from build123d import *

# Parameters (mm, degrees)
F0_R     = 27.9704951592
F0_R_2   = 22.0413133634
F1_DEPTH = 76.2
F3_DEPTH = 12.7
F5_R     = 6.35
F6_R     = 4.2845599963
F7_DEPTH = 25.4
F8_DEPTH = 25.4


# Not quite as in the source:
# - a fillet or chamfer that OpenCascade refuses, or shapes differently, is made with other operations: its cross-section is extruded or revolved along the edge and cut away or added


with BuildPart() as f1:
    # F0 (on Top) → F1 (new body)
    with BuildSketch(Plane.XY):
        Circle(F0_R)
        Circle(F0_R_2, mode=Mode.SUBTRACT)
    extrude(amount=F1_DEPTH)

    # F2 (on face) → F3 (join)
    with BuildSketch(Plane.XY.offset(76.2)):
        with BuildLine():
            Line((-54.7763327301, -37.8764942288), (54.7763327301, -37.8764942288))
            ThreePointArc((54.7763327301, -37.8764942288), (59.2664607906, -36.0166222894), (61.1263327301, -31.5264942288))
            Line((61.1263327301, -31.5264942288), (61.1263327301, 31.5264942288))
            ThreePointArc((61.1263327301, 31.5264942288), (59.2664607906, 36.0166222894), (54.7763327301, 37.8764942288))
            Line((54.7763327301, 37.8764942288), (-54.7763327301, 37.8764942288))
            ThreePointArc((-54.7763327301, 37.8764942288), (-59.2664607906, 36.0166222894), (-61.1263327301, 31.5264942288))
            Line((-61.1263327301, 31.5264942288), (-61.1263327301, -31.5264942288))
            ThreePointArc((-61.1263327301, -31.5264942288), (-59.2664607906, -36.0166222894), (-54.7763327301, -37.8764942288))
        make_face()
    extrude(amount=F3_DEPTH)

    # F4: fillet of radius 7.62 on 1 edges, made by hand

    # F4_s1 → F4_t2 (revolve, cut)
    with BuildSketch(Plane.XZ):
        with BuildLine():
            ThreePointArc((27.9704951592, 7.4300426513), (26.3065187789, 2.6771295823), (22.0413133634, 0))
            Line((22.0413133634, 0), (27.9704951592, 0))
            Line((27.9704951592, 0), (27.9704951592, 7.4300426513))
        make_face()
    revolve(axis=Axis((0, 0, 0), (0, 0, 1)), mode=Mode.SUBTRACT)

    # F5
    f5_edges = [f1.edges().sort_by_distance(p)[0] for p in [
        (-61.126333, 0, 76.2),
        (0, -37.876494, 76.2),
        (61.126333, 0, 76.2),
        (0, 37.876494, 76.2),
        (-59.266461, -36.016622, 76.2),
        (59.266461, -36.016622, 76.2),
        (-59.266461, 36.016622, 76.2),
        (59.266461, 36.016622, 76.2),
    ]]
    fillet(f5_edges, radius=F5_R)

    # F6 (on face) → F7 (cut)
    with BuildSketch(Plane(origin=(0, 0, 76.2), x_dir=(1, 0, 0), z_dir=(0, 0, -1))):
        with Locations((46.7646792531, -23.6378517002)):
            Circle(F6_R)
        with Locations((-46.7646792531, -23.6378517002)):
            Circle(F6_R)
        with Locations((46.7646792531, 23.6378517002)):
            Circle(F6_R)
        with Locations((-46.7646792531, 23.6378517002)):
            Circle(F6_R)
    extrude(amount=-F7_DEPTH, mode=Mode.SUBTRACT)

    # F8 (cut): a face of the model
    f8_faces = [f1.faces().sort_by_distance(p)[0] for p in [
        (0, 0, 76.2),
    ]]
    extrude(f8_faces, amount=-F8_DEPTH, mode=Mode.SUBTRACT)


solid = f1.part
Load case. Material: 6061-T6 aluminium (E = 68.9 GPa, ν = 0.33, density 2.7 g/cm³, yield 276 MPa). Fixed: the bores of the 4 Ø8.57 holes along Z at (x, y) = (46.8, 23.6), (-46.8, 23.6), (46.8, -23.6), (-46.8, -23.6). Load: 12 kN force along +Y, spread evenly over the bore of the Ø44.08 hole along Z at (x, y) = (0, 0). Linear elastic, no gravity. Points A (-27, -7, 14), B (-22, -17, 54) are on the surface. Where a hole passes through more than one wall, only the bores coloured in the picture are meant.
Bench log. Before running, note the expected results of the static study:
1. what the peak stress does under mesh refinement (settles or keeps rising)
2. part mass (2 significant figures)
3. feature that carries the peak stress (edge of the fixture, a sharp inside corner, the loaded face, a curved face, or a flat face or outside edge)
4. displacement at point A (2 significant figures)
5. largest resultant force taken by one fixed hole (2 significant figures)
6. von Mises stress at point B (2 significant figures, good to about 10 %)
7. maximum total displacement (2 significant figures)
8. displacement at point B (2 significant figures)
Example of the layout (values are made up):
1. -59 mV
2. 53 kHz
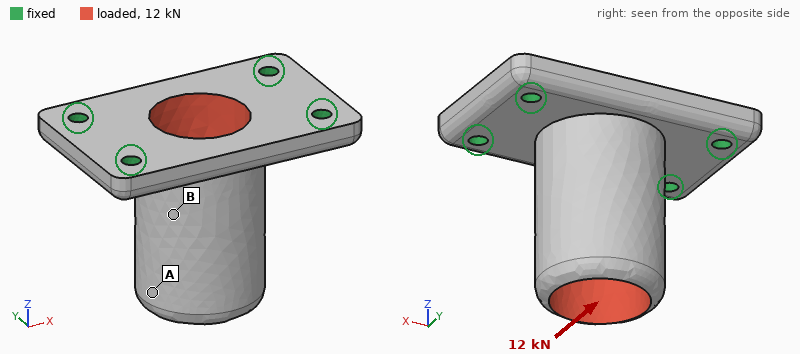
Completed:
1. keeps rising
2. 430 g
3. edge of the fixture
4. 0.23 mm
5. 5.9 kN
6. 21 MPa
7. 0.29 mm
8. 0.11 mm
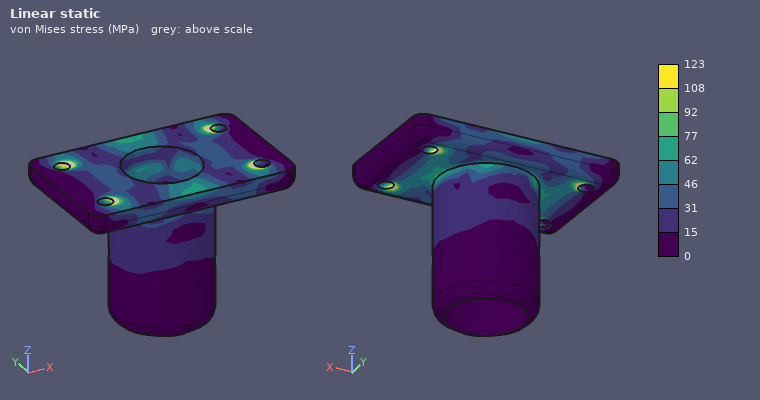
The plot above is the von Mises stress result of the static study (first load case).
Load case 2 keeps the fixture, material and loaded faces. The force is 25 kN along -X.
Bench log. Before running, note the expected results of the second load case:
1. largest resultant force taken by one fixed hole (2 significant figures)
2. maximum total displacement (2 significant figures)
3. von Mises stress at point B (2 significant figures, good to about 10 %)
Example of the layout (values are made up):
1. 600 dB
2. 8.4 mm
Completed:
1. 9.4 kN
2. 0.32 mm
3. 35 MPa
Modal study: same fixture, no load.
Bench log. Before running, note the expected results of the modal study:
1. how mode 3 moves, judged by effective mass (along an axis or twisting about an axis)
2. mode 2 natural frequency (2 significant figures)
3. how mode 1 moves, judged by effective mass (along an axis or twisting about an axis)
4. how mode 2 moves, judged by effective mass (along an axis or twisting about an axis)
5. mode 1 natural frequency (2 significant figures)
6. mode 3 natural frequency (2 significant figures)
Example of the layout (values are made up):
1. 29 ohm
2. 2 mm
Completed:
1. along Z
2. 3600 Hz
3. along Y
4. along X
5. 2600 Hz
6. 5300 Hz
